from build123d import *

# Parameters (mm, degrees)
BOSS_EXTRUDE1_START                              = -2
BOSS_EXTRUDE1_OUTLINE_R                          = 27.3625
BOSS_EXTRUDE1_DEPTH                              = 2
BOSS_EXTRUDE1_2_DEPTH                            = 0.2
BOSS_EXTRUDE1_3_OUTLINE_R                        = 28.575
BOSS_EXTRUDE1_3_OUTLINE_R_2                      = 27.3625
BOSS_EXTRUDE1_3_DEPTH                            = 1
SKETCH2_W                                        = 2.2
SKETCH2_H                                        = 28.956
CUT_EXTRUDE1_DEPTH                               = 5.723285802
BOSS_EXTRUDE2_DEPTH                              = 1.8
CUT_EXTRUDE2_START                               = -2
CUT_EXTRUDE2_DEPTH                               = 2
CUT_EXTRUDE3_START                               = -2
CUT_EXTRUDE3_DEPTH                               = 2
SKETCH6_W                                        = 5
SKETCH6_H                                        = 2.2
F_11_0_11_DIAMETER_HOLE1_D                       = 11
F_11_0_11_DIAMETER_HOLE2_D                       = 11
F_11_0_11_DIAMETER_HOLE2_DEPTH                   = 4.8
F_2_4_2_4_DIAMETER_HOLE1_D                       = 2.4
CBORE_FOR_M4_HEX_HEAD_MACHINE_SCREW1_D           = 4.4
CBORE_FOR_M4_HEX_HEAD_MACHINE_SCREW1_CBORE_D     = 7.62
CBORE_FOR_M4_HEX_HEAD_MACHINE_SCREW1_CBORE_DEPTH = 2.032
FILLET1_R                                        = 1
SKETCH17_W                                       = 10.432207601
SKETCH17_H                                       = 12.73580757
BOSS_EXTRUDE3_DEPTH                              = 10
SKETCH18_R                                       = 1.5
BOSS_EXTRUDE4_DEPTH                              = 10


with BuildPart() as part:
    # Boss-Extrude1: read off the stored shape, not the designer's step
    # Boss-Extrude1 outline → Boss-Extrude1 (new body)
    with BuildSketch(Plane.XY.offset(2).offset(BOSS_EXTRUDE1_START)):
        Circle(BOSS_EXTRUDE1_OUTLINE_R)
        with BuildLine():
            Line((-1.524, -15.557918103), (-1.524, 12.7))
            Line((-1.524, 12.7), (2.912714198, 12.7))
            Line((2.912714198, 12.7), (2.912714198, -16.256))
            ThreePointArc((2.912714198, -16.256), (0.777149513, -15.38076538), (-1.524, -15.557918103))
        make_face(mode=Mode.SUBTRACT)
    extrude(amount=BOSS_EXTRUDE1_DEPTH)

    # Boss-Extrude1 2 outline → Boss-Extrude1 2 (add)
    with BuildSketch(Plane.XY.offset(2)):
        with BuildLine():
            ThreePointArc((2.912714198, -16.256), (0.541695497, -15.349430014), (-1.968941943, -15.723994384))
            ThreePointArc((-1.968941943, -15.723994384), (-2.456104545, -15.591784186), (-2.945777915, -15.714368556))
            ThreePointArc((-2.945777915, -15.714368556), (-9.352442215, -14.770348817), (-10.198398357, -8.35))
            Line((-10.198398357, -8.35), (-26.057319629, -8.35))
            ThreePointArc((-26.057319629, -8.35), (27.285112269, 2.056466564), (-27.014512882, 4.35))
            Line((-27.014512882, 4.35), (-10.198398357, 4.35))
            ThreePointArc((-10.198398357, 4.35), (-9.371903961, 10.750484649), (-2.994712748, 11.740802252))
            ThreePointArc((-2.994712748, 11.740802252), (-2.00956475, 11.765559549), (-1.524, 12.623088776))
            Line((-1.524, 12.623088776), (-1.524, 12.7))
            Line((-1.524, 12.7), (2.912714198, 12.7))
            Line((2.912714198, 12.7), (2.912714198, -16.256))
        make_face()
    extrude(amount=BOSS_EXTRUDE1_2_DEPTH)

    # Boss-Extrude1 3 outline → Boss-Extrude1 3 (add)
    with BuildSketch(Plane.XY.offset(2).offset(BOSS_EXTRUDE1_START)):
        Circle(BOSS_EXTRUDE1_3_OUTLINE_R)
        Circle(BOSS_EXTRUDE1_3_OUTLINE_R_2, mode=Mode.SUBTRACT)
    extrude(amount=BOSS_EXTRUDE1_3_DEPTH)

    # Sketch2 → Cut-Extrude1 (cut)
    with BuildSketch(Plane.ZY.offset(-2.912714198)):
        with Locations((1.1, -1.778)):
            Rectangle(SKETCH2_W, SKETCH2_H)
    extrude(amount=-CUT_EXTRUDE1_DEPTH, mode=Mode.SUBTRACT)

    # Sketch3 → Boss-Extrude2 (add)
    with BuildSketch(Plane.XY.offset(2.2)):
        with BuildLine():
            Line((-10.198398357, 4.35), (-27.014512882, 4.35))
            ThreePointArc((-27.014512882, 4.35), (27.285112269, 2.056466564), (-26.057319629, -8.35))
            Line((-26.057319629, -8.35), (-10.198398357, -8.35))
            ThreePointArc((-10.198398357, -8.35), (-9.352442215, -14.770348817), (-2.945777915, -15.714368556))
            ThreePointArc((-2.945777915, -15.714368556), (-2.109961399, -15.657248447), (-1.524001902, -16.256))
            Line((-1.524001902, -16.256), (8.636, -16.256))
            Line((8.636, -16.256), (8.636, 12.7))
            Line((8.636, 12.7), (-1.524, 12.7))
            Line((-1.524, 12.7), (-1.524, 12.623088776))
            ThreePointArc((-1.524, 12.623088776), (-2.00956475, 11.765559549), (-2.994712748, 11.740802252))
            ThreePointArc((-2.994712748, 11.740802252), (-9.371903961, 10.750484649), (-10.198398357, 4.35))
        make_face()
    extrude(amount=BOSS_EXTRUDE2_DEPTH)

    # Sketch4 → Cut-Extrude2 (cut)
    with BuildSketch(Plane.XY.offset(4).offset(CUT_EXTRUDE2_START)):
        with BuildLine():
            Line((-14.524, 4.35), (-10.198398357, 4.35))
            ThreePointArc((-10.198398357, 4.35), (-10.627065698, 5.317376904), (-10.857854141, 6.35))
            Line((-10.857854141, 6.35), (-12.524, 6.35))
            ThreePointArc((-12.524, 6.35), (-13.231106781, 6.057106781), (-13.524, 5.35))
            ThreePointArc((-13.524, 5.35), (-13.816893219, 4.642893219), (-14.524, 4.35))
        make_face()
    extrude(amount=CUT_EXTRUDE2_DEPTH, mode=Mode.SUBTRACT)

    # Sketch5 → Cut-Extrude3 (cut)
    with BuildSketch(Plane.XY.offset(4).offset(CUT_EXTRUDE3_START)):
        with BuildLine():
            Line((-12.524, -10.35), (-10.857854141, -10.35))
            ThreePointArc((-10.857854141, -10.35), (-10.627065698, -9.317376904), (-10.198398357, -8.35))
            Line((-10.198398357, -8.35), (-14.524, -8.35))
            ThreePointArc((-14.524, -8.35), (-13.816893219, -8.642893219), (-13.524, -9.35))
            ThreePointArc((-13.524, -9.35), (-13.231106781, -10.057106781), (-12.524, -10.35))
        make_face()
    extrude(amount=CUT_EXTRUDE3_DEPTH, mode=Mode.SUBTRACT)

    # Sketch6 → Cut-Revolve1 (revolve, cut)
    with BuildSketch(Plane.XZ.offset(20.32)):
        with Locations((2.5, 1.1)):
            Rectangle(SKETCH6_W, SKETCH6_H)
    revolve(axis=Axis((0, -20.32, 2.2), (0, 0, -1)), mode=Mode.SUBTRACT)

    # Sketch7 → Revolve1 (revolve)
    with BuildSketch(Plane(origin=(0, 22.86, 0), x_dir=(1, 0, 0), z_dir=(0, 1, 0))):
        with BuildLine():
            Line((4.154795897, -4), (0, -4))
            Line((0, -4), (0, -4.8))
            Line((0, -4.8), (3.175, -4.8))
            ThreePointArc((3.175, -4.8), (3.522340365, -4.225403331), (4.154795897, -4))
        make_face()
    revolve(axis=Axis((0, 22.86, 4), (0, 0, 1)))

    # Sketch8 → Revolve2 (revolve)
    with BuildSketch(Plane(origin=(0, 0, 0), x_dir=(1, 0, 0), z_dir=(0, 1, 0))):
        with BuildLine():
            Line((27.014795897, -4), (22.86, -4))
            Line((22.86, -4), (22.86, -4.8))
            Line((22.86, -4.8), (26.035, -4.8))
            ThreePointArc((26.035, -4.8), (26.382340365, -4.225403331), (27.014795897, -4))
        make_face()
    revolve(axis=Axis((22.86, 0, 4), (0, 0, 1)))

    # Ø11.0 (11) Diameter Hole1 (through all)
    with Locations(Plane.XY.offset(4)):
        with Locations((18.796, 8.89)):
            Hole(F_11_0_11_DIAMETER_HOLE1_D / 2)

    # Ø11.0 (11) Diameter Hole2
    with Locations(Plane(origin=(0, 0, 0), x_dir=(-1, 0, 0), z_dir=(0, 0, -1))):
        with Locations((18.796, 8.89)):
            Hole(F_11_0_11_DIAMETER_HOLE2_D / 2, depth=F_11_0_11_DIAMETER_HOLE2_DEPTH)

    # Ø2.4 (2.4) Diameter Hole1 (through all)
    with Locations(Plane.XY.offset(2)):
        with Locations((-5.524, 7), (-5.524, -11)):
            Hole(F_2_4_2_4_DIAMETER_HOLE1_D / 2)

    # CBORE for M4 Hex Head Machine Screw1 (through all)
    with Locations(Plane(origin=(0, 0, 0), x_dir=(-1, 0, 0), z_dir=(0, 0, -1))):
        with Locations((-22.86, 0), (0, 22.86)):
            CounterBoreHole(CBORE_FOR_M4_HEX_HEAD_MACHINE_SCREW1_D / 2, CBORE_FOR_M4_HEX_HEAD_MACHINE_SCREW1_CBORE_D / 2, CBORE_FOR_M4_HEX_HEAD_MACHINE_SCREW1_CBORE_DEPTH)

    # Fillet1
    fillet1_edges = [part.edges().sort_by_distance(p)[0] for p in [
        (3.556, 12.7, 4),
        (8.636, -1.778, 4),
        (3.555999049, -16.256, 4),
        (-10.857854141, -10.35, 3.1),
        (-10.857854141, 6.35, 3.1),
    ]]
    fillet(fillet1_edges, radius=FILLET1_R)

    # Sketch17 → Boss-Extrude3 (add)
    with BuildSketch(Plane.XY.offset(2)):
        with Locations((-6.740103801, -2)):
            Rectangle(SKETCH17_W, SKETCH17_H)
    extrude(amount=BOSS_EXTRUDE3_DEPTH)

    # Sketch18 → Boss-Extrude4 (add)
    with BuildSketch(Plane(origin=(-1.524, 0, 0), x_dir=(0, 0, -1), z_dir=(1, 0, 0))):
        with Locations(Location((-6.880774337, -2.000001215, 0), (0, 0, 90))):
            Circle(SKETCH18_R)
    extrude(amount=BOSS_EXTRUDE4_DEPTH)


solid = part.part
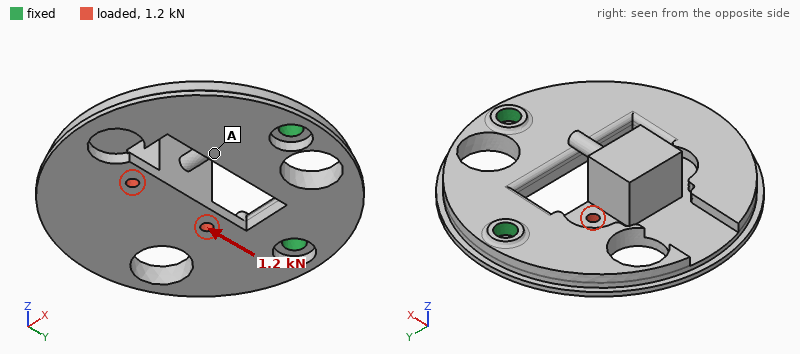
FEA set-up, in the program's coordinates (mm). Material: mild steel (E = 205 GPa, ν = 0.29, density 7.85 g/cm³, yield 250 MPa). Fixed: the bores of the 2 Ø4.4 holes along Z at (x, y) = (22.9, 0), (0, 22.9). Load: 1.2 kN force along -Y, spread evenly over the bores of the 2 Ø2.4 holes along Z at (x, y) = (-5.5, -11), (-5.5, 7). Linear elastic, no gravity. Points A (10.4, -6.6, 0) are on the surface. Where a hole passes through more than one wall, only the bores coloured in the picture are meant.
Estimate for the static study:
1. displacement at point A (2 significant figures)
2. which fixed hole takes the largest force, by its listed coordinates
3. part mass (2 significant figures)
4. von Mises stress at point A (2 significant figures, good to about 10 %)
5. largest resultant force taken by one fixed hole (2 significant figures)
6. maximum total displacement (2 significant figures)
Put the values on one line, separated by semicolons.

4.5 µm; (0, 22.9); 61 g; 16 MPa; 1.2 kN; 24 µm
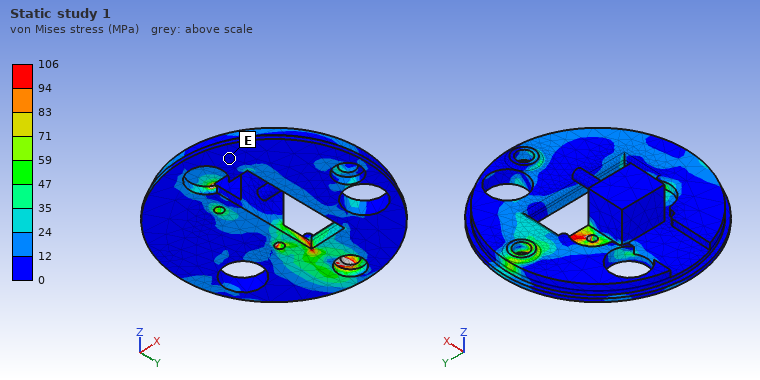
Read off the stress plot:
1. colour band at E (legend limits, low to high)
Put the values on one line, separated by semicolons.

0 to 12 MPa
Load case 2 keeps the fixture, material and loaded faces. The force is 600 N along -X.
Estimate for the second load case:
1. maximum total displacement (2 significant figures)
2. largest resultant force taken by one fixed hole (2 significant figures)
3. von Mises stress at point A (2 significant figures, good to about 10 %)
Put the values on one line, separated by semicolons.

25 µm; 390 N; 11 MPa
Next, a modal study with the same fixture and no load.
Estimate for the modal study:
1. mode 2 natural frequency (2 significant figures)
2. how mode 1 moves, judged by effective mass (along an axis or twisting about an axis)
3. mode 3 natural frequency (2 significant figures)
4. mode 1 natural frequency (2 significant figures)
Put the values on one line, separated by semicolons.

3400 Hz; along Z; 4900 Hz; 1400 Hz
